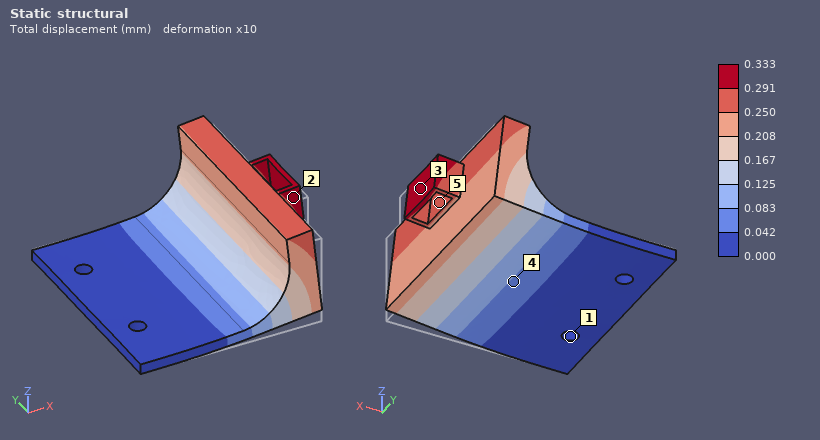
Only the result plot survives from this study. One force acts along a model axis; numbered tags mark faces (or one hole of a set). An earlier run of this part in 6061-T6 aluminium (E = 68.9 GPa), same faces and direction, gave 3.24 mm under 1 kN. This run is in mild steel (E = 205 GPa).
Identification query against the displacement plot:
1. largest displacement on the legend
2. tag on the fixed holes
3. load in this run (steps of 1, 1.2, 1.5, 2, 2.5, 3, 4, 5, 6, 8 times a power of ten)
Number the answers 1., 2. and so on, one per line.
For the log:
1. 0.333 mm
2. 1
3. 300 N
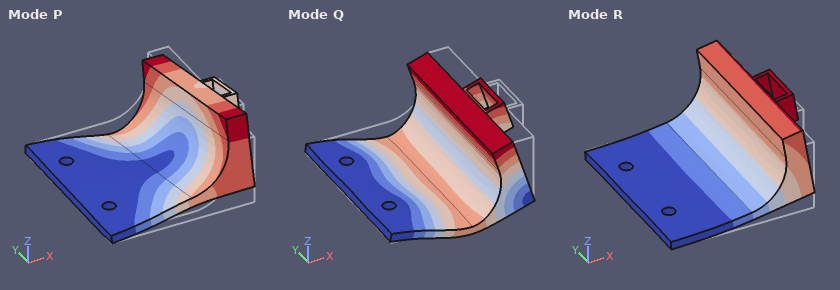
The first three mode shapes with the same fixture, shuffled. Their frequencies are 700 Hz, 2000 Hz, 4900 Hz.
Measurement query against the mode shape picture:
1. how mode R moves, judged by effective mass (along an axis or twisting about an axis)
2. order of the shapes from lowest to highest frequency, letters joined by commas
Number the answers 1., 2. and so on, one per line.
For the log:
1. along Z
2. R, P, Q
